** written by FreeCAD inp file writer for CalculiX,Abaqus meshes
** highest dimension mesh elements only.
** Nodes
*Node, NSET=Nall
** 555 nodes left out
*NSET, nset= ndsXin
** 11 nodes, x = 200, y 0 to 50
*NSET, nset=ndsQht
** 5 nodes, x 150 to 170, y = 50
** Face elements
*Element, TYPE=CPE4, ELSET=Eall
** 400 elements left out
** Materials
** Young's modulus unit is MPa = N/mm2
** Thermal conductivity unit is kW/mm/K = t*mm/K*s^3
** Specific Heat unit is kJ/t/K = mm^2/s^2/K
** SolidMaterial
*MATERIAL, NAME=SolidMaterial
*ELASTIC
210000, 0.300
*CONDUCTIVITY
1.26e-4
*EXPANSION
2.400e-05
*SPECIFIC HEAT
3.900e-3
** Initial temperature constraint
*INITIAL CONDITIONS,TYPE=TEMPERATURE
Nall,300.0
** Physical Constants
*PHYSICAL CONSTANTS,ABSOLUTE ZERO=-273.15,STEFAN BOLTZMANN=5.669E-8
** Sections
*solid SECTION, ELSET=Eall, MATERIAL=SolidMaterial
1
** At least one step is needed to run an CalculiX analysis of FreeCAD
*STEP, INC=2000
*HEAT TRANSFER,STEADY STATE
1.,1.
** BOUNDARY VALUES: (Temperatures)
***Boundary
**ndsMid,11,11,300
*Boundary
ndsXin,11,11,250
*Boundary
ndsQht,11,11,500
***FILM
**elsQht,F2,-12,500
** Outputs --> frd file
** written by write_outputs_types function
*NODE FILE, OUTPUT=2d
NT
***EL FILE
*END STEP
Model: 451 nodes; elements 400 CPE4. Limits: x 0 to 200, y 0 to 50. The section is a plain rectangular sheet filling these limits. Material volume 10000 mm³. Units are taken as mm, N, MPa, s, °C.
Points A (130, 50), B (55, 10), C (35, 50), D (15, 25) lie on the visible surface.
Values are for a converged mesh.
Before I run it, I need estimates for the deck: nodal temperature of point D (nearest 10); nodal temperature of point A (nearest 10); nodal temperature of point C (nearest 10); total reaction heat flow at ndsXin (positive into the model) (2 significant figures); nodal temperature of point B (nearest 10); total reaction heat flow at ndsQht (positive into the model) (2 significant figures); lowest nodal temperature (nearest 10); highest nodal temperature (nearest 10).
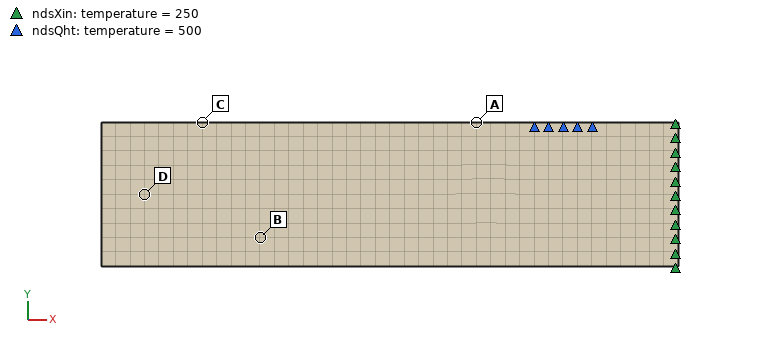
420 °C
430 °C
420 °C
-0.028 mW
420 °C
0.028 mW
250 °C
500 °C
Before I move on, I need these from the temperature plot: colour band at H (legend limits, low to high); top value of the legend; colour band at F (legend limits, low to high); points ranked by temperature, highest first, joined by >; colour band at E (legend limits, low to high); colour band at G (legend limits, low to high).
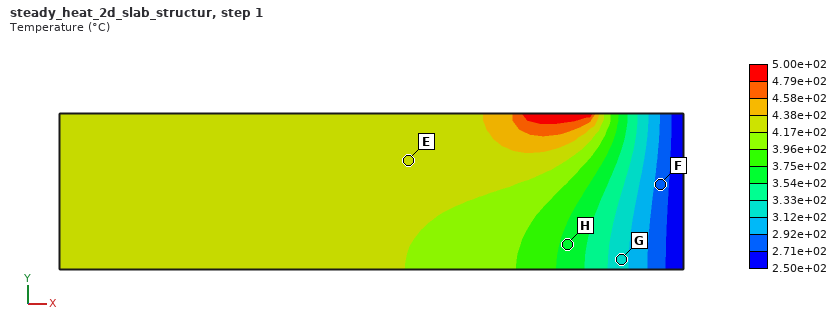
3.54e+02 to 3.75e+02 °C
5.00e+02 °C
2.71e+02 to 2.92e+02 °C
E > H > G > F
4.17e+02 to 4.38e+02 °C
3.12e+02 to 3.33e+02 °C
